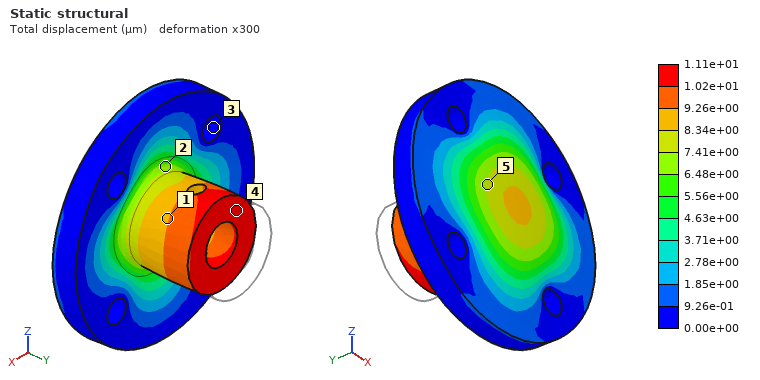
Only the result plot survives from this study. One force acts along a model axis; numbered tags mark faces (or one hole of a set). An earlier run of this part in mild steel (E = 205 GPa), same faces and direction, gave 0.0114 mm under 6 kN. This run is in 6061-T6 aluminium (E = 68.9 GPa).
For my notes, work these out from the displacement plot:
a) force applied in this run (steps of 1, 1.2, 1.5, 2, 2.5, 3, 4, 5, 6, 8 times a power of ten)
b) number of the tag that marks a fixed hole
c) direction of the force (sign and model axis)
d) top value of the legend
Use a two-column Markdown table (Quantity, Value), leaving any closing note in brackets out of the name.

| Quantity | Value |
|---|---|
| force applied in this run | 2 kN |
| number of the tag that marks a fixed hole | 3 |
| direction of the force | -Y |
| top value of the legend | 1.11e+01 µm |
